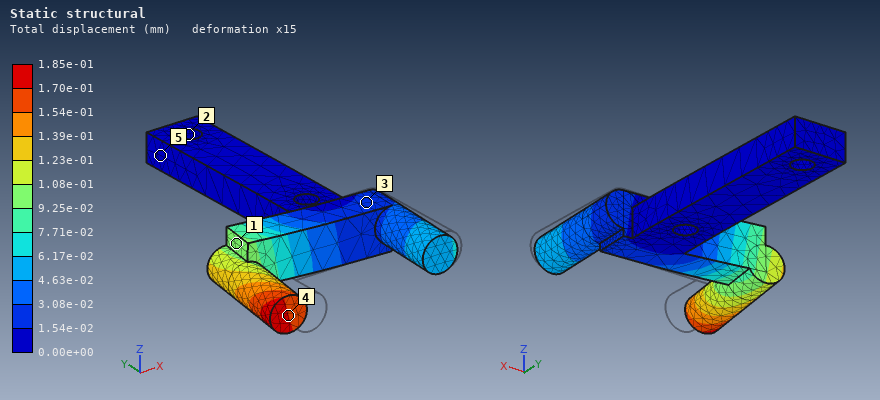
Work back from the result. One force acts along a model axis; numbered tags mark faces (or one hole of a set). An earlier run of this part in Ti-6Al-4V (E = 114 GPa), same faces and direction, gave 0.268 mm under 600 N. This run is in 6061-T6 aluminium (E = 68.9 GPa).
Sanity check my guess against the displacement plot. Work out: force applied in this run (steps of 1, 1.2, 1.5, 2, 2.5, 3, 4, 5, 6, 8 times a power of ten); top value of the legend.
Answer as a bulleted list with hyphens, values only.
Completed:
- 250 N
- 1.85e-01 mm
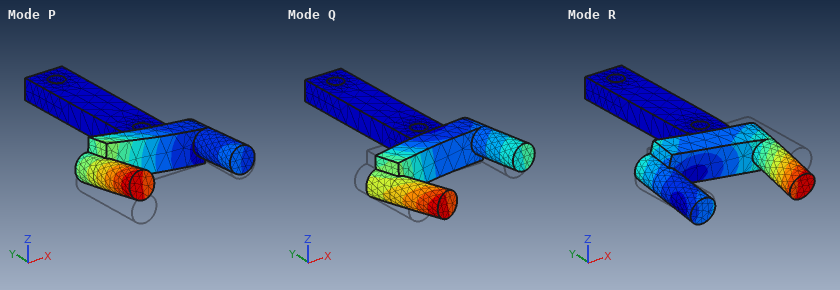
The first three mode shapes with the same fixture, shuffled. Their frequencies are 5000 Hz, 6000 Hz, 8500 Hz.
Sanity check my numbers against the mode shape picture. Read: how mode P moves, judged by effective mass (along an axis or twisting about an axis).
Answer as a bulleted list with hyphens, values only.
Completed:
- along Z
